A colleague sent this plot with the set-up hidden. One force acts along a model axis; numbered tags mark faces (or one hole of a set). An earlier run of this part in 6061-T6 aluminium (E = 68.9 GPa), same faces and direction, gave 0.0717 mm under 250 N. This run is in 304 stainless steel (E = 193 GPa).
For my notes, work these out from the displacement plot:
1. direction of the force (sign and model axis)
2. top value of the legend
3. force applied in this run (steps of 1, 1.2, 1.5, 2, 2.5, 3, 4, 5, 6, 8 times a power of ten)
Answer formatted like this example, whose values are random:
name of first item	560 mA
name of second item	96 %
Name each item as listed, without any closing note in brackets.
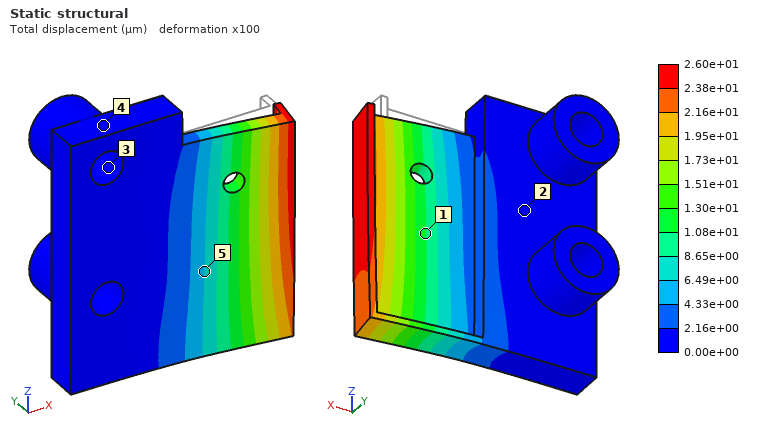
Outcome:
direction of the force	-Y
top value of the legend	2.60e+01 µm
force applied in this run	250 N
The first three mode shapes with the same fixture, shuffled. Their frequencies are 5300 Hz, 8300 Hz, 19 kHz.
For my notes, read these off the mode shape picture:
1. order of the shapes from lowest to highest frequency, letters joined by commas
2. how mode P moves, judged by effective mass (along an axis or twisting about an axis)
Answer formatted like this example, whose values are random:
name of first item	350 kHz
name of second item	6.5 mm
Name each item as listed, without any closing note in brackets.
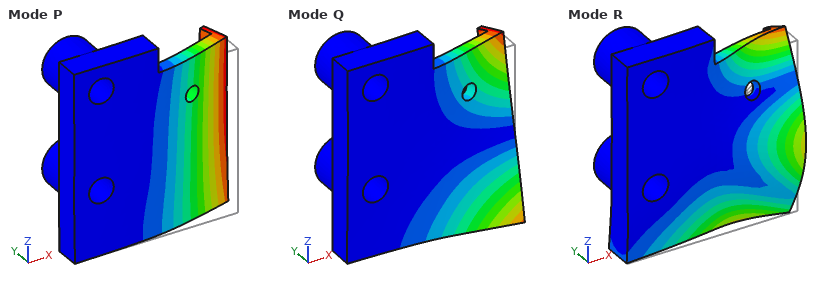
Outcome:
order of the shapes from lowest to highest frequency, letters joined by commas	P, Q, R
how mode P moves, judged by effective mass	along Y
